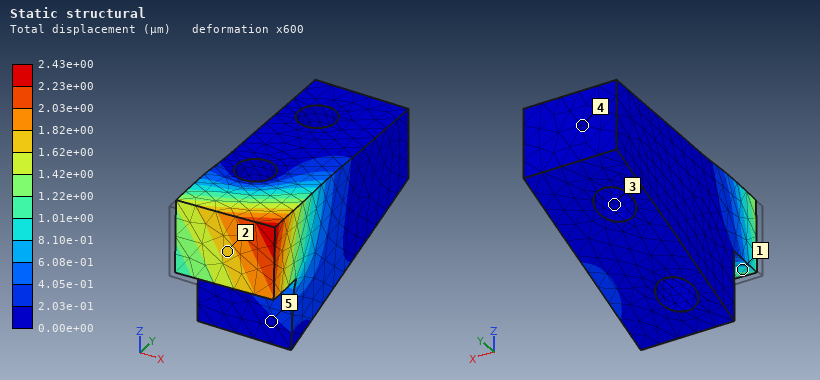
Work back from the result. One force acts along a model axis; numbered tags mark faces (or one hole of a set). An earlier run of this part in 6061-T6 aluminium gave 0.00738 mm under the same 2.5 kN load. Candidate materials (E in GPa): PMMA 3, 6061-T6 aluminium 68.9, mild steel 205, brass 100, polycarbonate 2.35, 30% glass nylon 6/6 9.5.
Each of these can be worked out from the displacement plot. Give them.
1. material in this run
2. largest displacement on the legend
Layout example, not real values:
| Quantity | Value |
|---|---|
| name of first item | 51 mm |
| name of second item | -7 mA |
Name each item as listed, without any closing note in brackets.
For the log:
| Quantity | Value |
|---|---|
| material in this run | mild steel |
| largest displacement on the legend | 2.43e+00 µm |
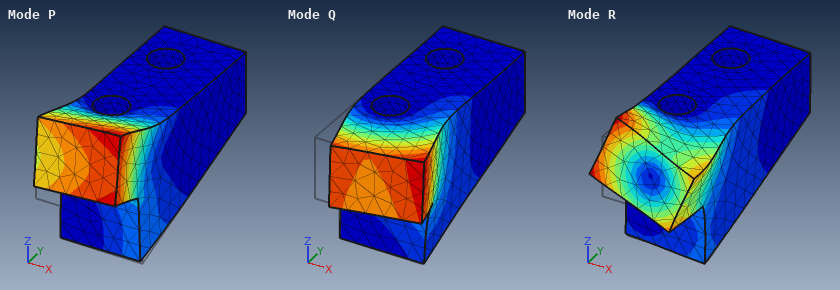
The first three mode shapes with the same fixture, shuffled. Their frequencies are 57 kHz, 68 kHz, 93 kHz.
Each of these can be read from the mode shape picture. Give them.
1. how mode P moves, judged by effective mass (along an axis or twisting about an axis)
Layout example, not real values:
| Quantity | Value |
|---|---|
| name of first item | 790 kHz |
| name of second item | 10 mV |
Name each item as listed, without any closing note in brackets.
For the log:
| Quantity | Value |
|---|---|
| how mode P moves, judged by effective mass | along Z |
